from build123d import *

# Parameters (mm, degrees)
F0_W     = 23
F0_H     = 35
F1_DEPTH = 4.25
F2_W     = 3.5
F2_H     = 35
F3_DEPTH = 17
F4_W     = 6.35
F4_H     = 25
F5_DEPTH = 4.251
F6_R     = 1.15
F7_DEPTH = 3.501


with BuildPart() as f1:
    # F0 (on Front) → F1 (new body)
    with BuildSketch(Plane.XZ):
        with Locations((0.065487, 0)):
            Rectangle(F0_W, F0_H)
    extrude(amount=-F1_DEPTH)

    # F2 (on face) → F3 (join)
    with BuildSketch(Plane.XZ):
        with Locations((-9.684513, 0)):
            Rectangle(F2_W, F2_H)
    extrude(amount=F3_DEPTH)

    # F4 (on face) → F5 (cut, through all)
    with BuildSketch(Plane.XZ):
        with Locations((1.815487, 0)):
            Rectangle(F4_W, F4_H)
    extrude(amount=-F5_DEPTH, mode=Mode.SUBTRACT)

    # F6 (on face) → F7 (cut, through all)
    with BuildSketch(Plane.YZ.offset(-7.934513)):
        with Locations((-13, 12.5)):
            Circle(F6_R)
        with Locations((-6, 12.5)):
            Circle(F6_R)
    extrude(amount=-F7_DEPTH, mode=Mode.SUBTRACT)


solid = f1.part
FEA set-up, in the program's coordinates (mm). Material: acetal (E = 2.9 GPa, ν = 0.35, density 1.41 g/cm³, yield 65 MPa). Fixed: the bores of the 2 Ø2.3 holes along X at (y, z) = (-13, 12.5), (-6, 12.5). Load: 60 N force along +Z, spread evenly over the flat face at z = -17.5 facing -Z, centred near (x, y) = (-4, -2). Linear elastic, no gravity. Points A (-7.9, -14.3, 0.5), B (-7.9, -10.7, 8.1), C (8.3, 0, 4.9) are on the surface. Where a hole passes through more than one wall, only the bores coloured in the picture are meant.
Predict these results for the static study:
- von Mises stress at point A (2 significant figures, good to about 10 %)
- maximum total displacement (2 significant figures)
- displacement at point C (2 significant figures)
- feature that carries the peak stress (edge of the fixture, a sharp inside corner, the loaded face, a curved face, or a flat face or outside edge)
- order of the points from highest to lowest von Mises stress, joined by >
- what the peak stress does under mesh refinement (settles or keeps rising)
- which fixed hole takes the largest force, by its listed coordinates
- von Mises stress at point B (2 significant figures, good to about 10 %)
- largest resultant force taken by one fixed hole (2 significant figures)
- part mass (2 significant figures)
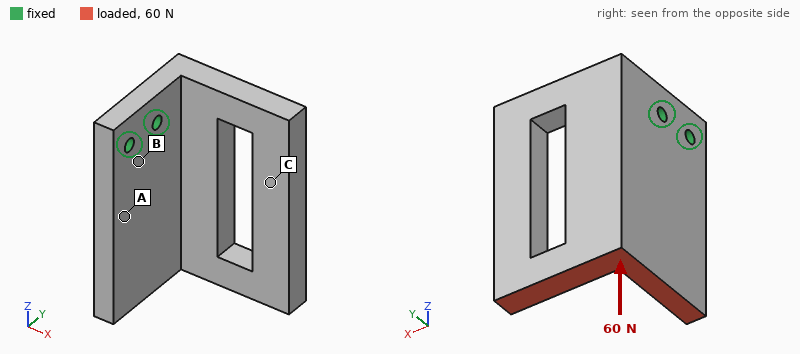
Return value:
2.5 MPa
0.42 mm
0.24 mm
edge of the fixture
B > A > C
keeps rising
(-6, 12.5)
4.8 MPa
81 N
6.8 g
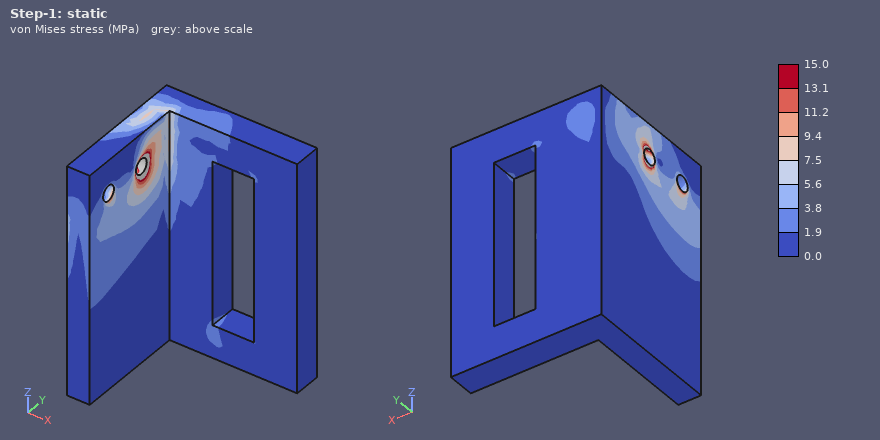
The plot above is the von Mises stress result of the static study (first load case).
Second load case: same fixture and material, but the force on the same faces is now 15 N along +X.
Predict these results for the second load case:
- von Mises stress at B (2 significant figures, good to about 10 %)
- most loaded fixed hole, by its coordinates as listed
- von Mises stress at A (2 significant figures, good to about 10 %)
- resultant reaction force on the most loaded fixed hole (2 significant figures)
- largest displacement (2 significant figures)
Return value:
6.4 MPa
(-6, 12.5)
3.3 MPa
17 N
0.49 mm
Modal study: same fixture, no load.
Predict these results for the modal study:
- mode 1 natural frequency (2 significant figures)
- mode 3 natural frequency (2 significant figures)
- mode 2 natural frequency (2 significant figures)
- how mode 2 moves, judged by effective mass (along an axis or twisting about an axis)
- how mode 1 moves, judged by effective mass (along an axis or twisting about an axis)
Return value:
620 Hz
1900 Hz
880 Hz
along Y
along X
